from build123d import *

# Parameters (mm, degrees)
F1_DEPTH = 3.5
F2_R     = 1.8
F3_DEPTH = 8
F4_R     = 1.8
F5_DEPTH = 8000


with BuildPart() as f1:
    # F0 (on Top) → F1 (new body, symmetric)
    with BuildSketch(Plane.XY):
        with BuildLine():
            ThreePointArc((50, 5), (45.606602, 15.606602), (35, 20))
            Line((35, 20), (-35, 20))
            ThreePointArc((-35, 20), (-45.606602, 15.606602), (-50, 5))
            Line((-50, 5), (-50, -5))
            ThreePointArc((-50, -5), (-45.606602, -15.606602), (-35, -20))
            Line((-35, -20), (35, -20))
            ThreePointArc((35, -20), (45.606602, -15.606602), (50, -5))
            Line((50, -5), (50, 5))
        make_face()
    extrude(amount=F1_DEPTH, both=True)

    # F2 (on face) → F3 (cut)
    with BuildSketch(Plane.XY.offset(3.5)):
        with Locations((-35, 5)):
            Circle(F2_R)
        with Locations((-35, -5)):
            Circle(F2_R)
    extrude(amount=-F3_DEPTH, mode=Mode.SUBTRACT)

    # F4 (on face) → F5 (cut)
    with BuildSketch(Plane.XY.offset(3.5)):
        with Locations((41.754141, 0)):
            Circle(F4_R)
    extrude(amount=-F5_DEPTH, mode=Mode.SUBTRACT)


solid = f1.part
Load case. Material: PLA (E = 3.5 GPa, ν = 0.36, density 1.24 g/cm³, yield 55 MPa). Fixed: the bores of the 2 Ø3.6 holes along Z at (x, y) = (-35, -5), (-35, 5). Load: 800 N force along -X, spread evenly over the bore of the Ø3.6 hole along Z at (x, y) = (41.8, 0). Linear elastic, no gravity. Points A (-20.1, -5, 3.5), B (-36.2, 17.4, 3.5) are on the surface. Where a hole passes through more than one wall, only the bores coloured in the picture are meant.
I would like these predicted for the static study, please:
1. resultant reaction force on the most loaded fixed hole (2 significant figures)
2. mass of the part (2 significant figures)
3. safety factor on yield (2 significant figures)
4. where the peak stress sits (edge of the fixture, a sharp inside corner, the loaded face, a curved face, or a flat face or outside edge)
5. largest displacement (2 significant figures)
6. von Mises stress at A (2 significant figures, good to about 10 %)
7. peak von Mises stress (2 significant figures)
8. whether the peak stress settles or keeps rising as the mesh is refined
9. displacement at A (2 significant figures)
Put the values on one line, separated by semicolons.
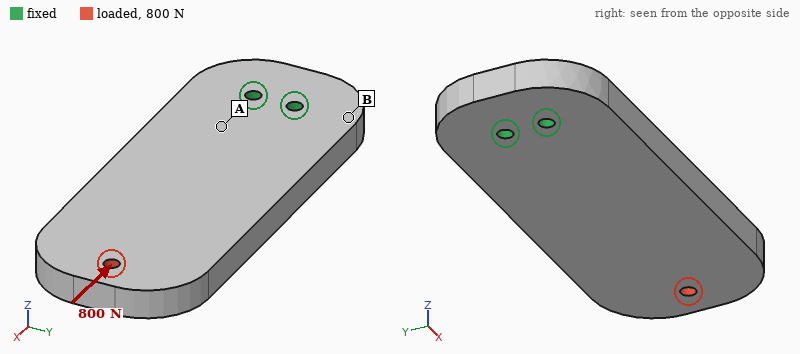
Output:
400 N; 33 g; 2.8; the loaded face; 97 µm; 3.7 MPa; 20 MPa; settles; 17 µm
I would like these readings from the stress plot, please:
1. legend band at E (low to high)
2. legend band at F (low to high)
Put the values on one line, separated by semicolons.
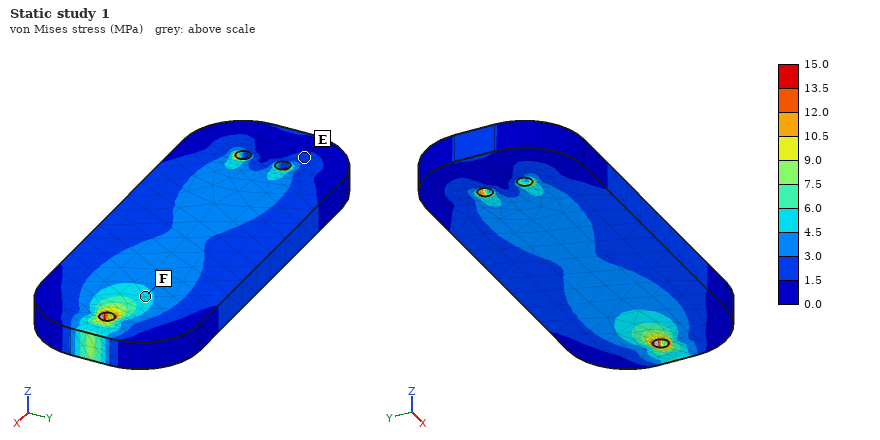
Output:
1.5 to 3.0 MPa; 4.5 to 6.0 MPa
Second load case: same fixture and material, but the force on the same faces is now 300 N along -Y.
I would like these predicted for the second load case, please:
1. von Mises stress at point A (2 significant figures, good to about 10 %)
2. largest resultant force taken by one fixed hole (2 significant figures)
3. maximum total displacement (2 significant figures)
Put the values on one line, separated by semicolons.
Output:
6.1 MPa; 1.8 kN; 1.1 mm
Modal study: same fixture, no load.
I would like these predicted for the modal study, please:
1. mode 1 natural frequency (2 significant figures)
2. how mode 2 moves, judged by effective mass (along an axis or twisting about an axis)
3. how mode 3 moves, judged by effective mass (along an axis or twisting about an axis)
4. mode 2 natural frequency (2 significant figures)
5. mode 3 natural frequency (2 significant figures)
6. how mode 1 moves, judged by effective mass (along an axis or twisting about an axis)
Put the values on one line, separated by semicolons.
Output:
270 Hz; along Y; twisting about X; 860 Hz; 1100 Hz; along Z
